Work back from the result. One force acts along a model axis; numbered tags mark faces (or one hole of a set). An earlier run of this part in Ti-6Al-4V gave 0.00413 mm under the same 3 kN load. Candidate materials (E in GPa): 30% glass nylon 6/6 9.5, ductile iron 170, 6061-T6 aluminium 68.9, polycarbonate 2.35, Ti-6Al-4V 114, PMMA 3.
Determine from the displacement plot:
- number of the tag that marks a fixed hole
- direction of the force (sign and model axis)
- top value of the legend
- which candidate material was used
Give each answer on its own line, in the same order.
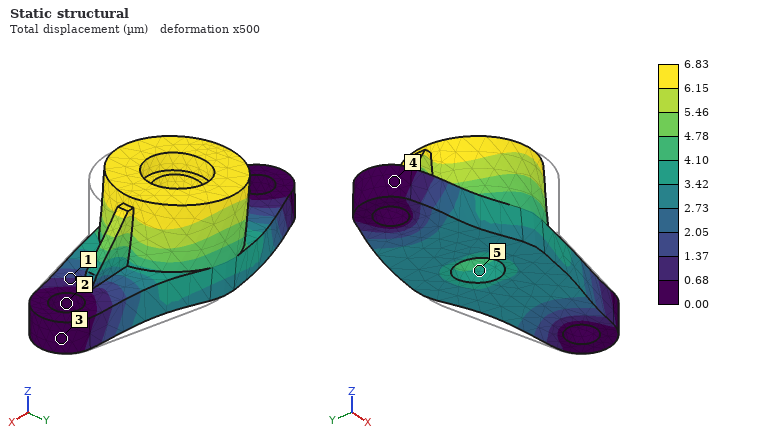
2
-X
6.83 µm
6061-T6 aluminium
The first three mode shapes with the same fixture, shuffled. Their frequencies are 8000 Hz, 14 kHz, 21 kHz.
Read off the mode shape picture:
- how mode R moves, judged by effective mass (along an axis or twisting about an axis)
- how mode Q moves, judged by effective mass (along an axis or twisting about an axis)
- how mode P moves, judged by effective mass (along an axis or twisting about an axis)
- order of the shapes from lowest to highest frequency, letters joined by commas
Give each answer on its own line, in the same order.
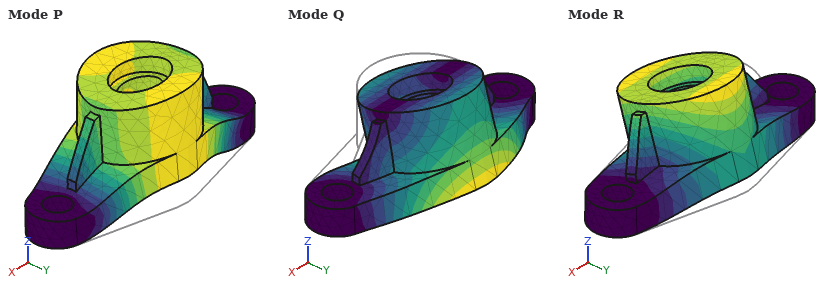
along Y
along Y
along Z
R, P, Q
